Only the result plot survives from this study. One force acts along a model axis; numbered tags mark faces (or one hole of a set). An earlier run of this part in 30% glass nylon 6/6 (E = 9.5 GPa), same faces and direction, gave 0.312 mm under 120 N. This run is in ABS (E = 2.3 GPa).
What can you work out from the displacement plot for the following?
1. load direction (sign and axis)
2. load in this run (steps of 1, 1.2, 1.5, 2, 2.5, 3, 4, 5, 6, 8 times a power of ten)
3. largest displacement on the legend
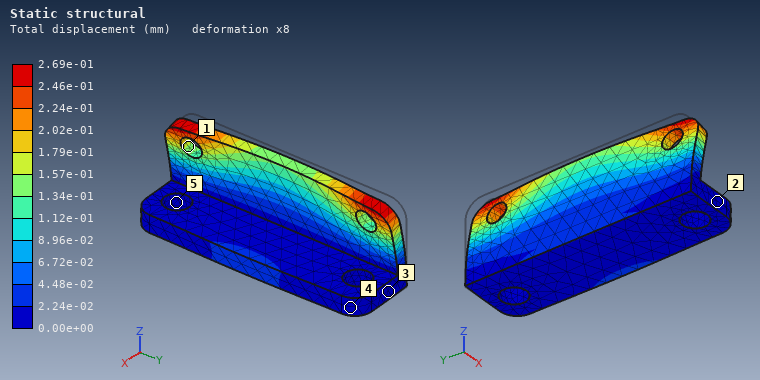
+X
25 N
2.69e-01 mm
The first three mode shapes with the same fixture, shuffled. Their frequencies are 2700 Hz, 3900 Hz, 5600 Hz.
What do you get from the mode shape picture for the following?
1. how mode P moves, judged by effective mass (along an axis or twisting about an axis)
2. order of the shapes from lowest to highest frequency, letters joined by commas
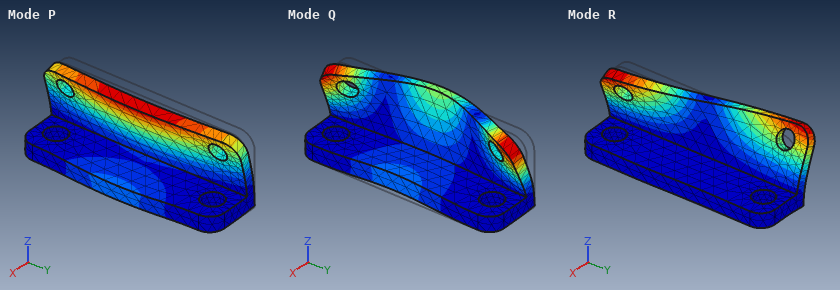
along X
P, R, Q
